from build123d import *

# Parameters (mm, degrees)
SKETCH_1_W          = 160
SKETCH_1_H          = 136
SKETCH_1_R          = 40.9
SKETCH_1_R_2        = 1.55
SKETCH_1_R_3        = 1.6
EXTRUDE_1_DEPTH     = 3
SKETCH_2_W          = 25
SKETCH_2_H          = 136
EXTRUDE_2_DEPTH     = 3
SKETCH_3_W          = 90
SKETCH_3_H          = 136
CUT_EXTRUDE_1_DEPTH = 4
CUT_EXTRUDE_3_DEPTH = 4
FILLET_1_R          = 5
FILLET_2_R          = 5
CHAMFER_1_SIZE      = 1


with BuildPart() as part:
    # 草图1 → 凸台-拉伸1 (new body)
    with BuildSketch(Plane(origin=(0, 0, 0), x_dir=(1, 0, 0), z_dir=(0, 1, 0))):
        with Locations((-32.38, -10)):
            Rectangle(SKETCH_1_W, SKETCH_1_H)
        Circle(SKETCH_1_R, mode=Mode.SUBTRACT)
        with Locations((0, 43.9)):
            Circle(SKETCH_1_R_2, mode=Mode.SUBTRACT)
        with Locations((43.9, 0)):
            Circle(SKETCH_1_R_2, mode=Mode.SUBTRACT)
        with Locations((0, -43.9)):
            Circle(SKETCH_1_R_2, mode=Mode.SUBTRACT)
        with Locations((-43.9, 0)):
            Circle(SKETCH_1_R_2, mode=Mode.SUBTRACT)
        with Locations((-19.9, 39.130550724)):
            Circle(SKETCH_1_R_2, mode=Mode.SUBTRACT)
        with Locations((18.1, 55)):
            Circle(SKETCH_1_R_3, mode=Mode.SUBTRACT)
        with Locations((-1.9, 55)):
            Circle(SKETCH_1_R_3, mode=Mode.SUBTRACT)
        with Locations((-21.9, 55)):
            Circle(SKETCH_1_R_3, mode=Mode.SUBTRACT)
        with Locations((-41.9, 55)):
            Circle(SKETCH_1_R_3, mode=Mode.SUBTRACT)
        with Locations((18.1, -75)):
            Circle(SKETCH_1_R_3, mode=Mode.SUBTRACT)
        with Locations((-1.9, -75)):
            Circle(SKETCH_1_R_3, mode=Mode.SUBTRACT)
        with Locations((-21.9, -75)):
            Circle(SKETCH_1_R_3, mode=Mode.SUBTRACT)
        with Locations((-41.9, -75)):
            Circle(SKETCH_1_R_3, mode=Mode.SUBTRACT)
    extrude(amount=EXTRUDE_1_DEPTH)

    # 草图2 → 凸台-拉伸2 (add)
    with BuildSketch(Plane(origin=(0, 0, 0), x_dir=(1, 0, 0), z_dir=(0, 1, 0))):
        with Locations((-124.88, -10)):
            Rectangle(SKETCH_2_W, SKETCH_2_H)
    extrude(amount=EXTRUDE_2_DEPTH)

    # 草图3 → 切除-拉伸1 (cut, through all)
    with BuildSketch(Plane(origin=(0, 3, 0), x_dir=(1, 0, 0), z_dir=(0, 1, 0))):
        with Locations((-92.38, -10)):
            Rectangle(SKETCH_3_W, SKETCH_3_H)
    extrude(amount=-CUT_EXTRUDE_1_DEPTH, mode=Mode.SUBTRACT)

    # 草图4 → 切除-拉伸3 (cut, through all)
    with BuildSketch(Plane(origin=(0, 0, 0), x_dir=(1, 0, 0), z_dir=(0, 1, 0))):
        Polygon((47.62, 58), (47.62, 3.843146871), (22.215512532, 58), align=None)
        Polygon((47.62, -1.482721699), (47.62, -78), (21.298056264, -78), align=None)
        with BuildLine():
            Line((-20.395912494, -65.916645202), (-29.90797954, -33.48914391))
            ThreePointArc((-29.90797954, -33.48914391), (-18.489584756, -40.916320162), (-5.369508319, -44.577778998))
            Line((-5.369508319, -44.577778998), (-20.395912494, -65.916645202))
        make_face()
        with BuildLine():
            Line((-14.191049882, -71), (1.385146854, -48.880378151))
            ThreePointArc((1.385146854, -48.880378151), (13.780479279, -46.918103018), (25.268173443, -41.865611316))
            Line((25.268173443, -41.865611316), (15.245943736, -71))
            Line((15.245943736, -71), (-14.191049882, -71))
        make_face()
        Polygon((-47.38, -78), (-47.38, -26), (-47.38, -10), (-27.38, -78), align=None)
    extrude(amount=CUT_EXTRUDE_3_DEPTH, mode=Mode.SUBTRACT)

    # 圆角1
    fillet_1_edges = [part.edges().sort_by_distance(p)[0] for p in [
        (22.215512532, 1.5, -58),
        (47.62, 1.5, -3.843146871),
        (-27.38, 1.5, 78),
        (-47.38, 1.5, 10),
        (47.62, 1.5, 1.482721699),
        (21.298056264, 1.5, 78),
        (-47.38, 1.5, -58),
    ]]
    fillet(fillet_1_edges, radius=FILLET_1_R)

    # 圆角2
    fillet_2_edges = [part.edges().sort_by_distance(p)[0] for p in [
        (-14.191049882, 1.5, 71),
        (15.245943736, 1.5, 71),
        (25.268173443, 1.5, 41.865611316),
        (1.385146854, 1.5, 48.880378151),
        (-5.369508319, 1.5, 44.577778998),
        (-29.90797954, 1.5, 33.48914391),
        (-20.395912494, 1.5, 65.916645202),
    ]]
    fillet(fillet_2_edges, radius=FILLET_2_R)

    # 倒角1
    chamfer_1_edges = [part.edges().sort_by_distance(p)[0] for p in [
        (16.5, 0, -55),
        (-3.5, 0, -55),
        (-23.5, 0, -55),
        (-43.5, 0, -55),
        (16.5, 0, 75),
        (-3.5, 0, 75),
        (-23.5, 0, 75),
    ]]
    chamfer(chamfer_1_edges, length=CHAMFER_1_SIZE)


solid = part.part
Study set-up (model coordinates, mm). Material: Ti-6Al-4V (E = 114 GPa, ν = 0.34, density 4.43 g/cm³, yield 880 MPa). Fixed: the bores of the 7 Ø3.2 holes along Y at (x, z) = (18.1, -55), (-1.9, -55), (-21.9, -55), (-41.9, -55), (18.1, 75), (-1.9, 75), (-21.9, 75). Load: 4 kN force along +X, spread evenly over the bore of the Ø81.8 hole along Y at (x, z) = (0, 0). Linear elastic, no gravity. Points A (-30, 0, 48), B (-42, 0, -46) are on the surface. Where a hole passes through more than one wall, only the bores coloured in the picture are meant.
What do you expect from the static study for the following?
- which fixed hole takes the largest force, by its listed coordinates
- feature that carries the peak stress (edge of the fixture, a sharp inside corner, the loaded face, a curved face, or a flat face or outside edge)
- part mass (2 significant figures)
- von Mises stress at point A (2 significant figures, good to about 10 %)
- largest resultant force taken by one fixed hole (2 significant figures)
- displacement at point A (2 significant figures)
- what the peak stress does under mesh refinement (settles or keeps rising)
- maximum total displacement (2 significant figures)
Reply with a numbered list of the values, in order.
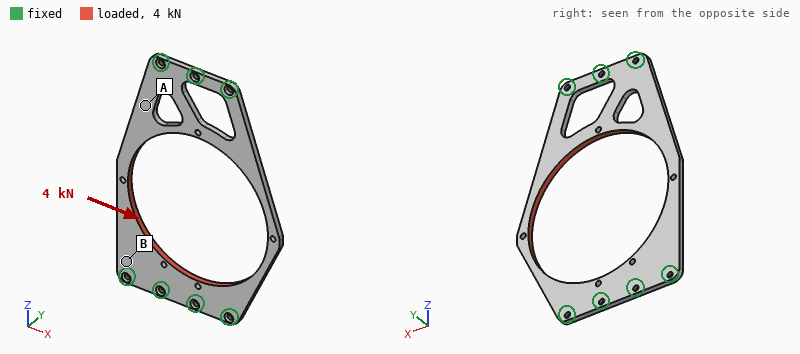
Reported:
1. (-1.9, 75)
2. edge of the fixture
3. 58 g
4. 41 MPa
5. 1.2 kN
6. 0.054 mm
7. keeps rising
8. 0.10 mm
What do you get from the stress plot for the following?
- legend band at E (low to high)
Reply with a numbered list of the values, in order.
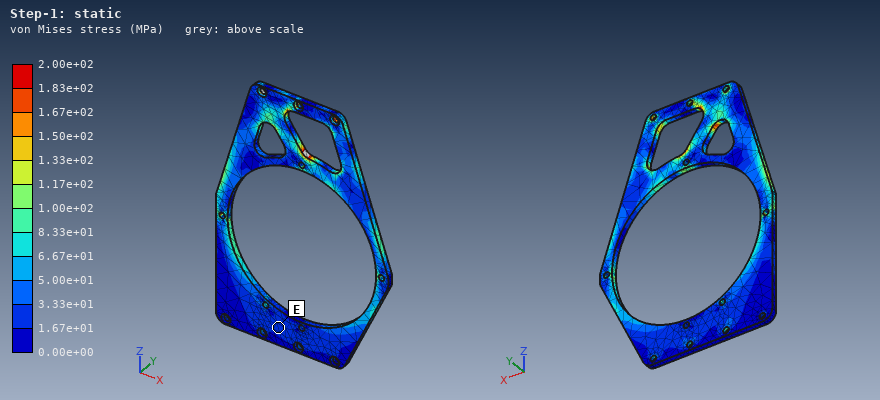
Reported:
1. 1.67e+01 to 3.33e+01 MPa
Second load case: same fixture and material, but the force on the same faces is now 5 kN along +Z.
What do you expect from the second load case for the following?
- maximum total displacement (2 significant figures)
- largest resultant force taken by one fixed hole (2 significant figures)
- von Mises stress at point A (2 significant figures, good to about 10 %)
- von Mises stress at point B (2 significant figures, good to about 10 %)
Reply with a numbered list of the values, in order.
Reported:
1. 72 µm
2. 1.3 kN
3. 25 MPa
4. 19 MPa
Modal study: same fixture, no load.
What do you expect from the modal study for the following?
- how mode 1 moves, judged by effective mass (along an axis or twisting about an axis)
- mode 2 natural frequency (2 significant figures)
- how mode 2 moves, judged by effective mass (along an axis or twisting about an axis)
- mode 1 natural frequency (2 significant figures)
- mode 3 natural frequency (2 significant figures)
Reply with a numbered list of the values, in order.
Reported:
1. along Y
2. 1100 Hz
3. along Y
4. 900 Hz
5. 2000 Hz
